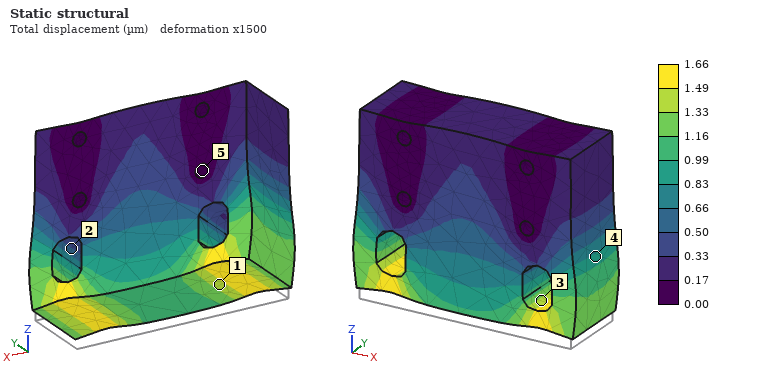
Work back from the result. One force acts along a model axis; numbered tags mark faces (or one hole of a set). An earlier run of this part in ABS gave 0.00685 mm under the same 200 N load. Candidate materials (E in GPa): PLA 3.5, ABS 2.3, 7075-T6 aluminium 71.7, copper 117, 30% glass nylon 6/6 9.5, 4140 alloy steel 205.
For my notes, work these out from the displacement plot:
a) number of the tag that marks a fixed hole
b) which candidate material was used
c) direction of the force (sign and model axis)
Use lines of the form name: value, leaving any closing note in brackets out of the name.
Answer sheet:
number of the tag that marks a fixed hole: 5
which candidate material was used: 30% glass nylon 6/6
direction of the force: +Z
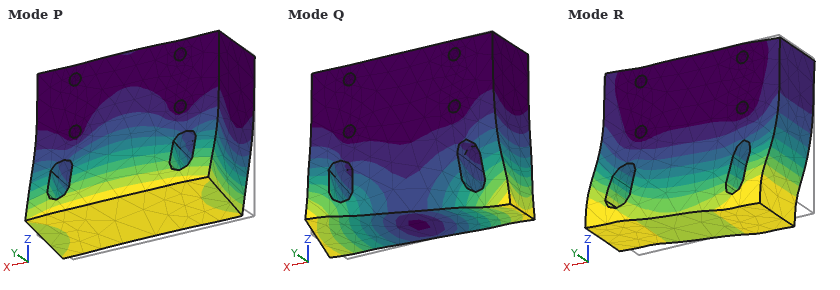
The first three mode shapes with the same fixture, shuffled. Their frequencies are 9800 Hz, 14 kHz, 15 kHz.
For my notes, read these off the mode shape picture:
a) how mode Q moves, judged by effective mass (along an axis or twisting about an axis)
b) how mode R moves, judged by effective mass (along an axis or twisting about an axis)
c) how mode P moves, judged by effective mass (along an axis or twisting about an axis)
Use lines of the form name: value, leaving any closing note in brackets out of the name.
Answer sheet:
how mode Q moves, judged by effective mass: twisting about Z
how mode R moves, judged by effective mass: along X
how mode P moves, judged by effective mass: along Y
